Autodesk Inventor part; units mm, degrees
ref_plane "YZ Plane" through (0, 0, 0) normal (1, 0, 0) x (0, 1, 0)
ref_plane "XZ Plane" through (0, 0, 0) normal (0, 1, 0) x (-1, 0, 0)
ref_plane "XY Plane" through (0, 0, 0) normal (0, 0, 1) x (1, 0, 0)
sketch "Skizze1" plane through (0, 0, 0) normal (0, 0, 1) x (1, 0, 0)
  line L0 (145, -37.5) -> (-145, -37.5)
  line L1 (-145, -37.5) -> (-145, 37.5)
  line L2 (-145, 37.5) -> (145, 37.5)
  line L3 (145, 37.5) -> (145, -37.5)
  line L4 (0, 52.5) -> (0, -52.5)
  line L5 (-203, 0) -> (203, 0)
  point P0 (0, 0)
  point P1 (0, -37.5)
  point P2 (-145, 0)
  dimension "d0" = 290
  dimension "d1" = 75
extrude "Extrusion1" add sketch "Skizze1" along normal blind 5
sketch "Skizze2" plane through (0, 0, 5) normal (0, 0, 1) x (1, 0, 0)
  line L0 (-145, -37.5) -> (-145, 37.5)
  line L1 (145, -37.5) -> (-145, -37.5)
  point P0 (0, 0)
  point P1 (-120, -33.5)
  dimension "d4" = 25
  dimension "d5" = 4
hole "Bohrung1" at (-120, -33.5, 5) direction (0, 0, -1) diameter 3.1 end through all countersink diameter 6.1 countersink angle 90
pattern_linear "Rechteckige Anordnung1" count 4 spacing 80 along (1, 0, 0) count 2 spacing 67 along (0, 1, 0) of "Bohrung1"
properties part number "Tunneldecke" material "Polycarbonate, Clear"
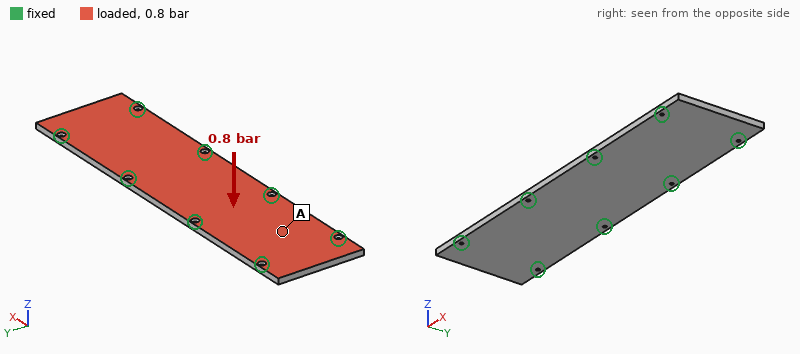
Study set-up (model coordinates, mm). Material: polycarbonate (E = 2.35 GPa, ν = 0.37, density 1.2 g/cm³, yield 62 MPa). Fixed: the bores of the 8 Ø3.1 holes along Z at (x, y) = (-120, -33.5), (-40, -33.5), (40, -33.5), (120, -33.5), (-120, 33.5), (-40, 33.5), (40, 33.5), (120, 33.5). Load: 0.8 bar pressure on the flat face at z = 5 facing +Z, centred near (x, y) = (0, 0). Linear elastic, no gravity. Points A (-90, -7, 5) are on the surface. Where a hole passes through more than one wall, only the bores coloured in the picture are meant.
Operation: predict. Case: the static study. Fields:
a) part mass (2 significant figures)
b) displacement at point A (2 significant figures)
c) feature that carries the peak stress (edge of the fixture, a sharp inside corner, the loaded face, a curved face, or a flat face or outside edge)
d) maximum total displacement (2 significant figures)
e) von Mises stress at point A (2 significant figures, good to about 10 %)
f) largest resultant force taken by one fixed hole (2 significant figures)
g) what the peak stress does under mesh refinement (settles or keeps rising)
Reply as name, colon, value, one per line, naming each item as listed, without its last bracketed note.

part mass: 130 g
displacement at point A: 0.71 mm
feature that carries the peak stress: edge of the fixture
maximum total displacement: 0.76 mm
von Mises stress at point A: 5.5 MPa
largest resultant force taken by one fixed hole: 260 N
what the peak stress does under mesh refinement: keeps rising
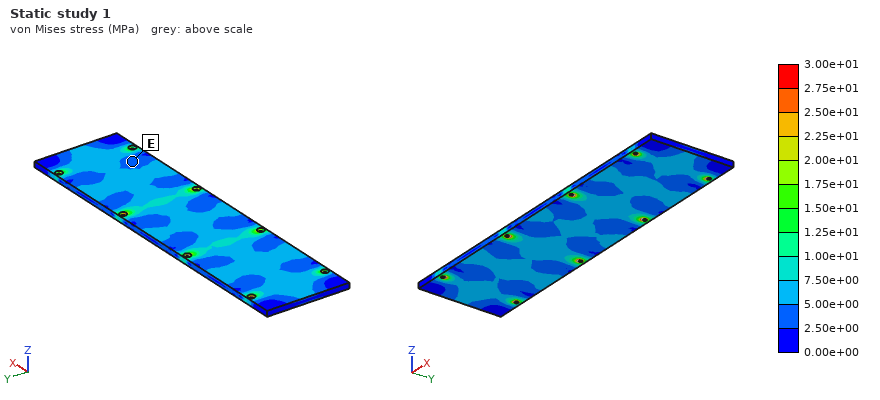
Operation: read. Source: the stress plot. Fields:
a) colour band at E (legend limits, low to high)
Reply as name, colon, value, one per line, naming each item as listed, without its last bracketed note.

colour band at E: 2.50e+00 to 5.00e+00 MPa
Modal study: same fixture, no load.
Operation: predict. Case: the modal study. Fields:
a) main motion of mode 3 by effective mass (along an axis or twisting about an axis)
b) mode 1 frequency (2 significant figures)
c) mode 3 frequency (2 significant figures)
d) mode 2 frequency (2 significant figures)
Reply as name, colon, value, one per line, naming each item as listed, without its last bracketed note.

main motion of mode 3 by effective mass: along Z
mode 1 frequency: 710 Hz
mode 3 frequency: 780 Hz
mode 2 frequency: 740 Hz
